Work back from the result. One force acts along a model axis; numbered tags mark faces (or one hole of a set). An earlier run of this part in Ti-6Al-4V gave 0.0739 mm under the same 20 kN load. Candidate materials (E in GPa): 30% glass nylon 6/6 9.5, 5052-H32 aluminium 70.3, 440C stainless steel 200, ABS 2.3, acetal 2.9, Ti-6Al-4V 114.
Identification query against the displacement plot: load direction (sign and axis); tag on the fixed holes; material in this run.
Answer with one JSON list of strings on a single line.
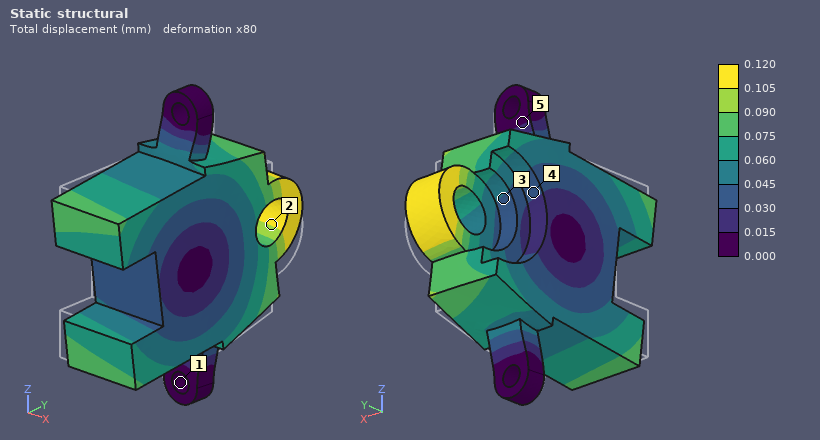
["+Z", "1", "5052-H32 aluminium"]
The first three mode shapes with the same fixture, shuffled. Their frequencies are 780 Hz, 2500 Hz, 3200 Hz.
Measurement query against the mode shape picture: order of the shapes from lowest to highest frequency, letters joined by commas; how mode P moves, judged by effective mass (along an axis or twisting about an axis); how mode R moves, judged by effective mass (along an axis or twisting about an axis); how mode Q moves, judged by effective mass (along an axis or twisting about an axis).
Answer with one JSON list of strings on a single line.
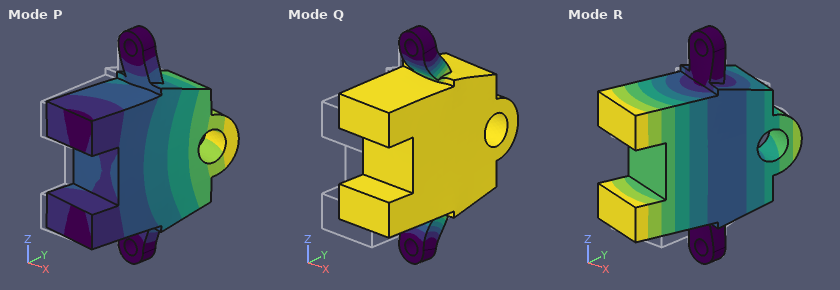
["R, Q, P", "along X", "along X", "along Y"]
